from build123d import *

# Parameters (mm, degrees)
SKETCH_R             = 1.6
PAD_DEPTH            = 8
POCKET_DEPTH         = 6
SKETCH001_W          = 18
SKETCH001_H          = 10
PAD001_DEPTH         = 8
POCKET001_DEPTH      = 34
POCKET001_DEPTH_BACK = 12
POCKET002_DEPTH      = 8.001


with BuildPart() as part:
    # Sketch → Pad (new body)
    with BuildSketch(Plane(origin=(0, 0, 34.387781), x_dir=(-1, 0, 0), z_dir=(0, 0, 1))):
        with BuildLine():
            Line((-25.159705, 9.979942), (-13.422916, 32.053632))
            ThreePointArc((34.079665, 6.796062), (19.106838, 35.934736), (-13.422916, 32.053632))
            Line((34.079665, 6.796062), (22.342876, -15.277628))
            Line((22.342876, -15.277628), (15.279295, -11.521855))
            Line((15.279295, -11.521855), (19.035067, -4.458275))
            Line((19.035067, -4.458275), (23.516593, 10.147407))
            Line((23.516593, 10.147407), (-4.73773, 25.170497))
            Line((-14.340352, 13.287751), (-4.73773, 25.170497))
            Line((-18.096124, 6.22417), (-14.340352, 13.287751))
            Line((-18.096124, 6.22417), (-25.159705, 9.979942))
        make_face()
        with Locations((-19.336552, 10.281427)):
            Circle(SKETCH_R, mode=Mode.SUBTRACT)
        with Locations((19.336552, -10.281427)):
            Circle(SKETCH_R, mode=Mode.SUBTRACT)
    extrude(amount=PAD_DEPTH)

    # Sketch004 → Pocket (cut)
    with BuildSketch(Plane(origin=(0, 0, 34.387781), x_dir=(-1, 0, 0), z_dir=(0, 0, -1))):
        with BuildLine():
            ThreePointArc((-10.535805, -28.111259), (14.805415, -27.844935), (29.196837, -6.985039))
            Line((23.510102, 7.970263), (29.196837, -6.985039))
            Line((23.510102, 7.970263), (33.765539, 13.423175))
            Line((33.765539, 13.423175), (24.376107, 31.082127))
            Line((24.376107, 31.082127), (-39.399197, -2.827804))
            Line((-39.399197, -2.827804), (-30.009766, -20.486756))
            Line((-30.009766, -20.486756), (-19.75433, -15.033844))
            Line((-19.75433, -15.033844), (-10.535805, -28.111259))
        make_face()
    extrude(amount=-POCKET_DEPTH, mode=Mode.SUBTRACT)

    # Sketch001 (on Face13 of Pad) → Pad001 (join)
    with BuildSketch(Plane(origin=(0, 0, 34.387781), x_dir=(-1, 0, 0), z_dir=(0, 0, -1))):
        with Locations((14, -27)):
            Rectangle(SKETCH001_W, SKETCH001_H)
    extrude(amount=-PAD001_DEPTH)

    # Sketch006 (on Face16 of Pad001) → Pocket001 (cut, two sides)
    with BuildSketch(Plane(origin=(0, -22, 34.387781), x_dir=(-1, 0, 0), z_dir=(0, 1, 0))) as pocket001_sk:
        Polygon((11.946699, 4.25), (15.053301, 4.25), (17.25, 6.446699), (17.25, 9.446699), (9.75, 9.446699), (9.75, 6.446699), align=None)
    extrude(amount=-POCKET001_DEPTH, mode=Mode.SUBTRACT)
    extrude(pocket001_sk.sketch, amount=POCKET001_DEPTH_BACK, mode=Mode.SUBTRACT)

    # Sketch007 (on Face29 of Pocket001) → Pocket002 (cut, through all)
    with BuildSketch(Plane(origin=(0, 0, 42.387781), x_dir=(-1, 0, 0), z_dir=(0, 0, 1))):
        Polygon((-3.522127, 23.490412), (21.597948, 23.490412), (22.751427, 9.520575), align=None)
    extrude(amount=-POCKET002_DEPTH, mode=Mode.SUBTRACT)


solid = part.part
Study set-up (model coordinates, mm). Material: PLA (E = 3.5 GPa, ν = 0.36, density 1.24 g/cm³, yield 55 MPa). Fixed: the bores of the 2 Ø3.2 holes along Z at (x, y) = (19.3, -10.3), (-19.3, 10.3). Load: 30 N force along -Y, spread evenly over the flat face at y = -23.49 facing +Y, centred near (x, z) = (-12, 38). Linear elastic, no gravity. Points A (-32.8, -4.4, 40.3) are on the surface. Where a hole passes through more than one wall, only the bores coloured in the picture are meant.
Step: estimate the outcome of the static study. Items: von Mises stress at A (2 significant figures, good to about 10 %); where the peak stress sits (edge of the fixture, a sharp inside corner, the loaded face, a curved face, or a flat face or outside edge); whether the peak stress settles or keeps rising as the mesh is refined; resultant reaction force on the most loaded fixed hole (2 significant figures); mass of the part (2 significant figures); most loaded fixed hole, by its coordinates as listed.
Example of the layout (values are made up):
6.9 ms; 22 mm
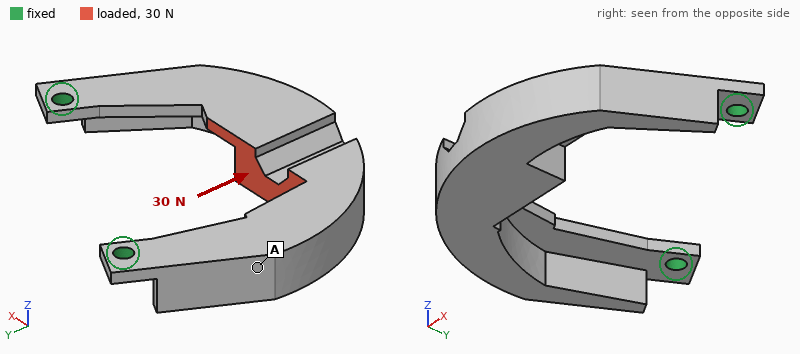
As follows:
1.3 MPa; edge of the fixture; keeps rising; 21 N; 7.2 g; (-19.3, 10.3)
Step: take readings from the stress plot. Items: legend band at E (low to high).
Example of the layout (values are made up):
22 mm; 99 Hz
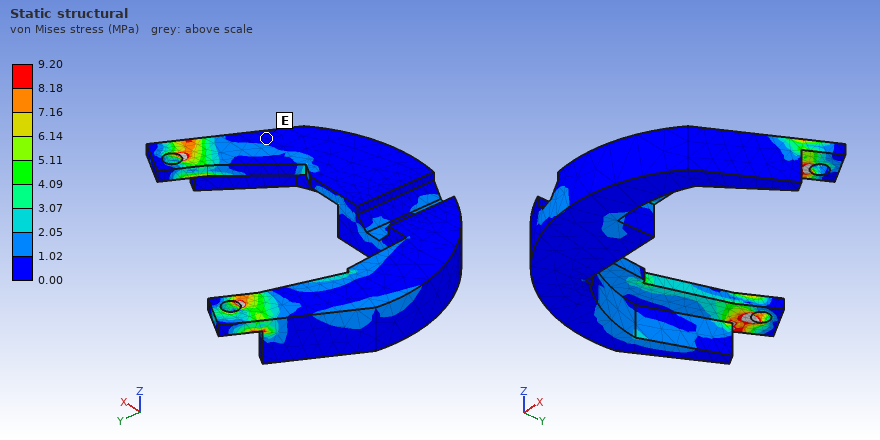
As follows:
0.00 to 1.02 MPa
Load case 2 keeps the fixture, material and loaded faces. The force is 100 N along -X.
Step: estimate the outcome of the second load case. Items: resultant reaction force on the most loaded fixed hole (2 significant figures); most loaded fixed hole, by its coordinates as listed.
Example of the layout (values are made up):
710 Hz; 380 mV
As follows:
82 N; (19.3, -10.3)
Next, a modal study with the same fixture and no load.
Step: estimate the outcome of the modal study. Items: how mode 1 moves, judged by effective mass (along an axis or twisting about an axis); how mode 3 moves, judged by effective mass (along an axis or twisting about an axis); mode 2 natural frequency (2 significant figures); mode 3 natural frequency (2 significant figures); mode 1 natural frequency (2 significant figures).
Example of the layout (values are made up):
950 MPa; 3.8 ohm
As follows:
along Z; along X; 1000 Hz; 1400 Hz; 210 Hz
